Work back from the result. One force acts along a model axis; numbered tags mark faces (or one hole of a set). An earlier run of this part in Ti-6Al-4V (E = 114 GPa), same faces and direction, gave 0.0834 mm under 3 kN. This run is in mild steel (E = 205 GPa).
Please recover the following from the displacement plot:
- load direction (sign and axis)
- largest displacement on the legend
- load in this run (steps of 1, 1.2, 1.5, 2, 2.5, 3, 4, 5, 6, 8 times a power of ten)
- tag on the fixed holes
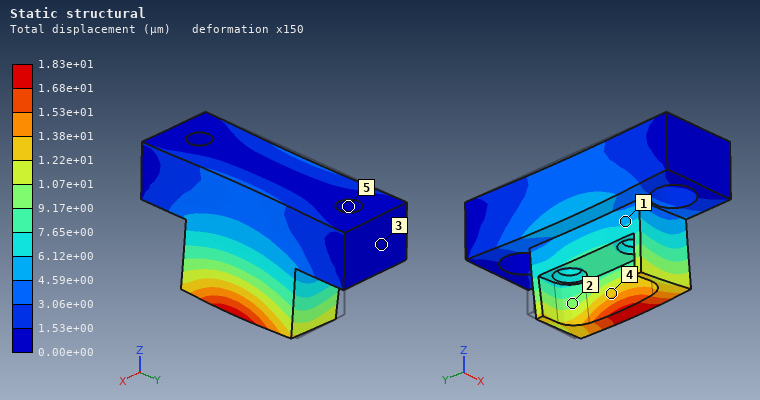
+X
1.83e+01 µm
1.2 kN
5
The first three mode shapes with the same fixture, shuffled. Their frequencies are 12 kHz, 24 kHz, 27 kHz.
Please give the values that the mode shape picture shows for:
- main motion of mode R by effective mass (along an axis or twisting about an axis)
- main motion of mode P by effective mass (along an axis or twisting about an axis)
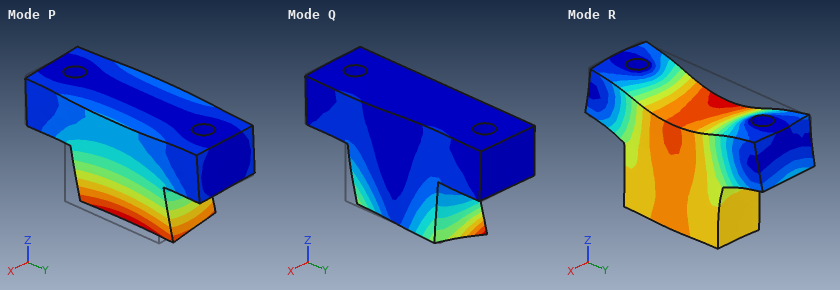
along Z
along X
